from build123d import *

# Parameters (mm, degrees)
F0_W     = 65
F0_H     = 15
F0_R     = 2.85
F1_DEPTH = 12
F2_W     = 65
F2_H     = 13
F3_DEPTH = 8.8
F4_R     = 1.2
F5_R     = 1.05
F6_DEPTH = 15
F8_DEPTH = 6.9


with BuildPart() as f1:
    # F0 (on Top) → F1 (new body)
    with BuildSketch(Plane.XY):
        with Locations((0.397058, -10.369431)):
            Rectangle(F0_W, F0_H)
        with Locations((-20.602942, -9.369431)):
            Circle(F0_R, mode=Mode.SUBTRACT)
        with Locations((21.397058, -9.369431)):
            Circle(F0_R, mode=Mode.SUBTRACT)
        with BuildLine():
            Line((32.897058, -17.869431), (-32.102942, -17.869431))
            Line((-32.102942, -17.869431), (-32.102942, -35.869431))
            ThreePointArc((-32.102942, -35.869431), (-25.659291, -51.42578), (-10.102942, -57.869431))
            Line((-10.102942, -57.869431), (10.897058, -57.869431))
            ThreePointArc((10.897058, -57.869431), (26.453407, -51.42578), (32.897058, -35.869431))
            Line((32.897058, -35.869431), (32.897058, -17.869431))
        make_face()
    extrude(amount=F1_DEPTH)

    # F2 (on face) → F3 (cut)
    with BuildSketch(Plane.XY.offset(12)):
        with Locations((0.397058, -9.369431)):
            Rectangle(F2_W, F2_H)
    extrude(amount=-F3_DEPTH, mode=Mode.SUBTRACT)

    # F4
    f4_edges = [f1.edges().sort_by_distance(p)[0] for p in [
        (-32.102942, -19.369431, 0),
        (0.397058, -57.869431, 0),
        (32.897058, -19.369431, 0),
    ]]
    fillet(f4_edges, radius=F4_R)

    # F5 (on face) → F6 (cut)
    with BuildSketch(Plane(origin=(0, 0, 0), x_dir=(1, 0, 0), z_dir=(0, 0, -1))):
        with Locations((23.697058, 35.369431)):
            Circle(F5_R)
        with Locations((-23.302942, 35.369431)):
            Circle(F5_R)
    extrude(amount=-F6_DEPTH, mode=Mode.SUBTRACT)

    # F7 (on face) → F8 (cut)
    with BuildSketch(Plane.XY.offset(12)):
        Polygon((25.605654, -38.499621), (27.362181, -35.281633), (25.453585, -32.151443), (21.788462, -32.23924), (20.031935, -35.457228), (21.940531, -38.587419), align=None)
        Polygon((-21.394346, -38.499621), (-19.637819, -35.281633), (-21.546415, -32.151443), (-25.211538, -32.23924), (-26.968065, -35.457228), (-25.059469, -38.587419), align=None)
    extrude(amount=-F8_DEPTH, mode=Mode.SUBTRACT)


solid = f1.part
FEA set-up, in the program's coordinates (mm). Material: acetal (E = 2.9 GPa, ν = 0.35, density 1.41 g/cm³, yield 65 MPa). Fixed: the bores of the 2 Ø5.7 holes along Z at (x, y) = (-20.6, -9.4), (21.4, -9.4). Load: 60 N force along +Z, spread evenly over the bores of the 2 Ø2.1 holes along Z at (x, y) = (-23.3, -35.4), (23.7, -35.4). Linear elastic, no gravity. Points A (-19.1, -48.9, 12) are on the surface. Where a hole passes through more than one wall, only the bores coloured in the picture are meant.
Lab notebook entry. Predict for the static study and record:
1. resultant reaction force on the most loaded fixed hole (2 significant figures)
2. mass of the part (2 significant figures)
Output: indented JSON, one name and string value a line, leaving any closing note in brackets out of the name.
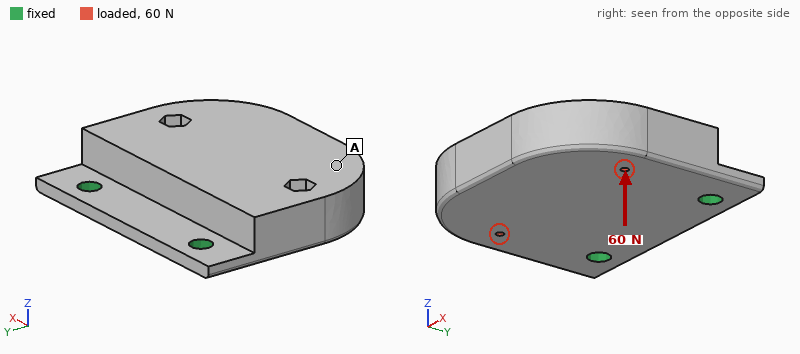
{
  "resultant reaction force on the most loaded fixed hole": "30 N",
  "mass of the part": "45 g"
}
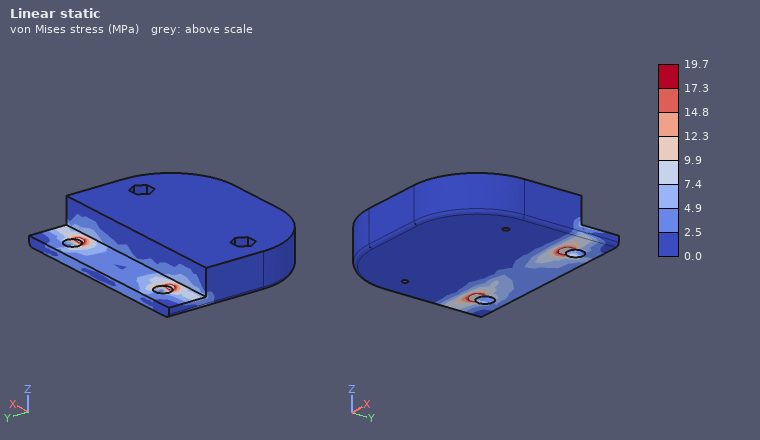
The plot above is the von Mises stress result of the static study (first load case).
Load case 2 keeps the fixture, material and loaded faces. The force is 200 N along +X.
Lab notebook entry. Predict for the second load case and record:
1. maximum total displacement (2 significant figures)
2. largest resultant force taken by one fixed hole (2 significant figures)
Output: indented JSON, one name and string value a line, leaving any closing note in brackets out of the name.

{
  "maximum total displacement": "47 µm",
  "largest resultant force taken by one fixed hole": "150 N"
}
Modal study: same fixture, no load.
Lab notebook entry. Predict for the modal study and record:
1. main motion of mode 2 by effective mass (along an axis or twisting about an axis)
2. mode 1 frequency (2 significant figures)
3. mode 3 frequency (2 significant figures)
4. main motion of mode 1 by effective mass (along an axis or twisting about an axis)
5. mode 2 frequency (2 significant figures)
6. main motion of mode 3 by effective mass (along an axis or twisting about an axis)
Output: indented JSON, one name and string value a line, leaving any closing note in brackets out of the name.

{
  "main motion of mode 2 by effective mass": "twisting about Y",
  "mode 1 frequency": "240 Hz",
  "mode 3 frequency": "2100 Hz",
  "main motion of mode 1 by effective mass": "along Z",
  "mode 2 frequency": "1500 Hz",
  "main motion of mode 3 by effective mass": "along X"
}
